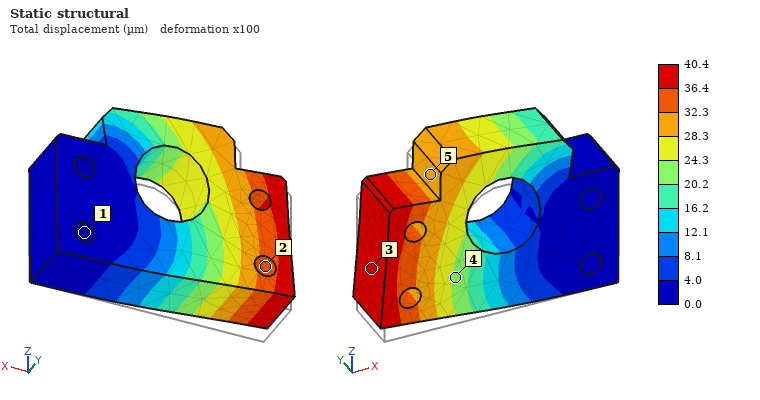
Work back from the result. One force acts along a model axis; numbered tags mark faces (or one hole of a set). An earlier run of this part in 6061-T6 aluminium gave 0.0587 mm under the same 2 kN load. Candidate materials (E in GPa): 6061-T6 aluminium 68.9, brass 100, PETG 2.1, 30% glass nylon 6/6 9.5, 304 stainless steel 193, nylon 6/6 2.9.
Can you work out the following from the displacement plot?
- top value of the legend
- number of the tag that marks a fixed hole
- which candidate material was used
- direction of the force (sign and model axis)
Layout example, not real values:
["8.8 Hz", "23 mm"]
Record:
["40.4 µm", "1", "brass", "+Z"]
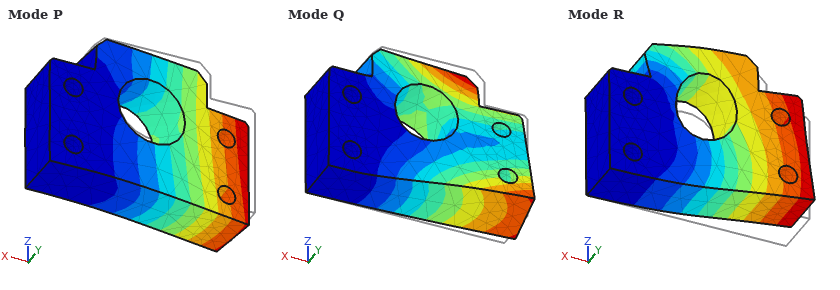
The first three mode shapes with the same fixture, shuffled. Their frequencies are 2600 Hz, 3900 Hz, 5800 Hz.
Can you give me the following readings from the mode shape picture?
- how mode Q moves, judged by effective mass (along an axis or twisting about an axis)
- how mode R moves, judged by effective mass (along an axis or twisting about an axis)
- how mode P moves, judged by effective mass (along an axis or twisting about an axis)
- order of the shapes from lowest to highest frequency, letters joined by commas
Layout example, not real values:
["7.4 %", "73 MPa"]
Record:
["twisting about X", "along Z", "along Y", "P, R, Q"]
